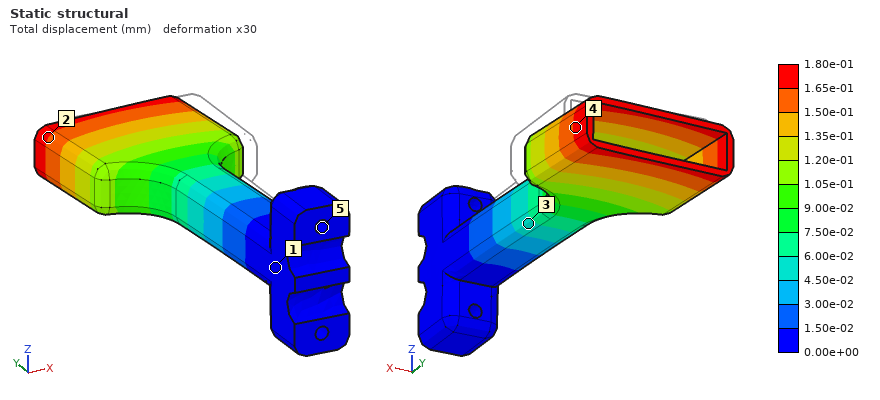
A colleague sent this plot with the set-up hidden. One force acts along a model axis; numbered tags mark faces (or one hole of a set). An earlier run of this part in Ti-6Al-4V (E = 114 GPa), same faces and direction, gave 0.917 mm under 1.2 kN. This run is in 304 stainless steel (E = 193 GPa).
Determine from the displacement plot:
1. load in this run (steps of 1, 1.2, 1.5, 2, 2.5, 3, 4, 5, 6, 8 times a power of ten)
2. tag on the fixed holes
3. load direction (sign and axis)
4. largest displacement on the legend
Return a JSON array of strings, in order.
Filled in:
["400 N", "5", "-X", "1.80e-01 mm"]
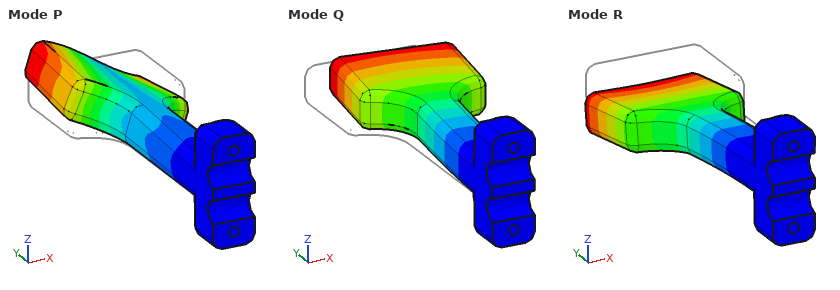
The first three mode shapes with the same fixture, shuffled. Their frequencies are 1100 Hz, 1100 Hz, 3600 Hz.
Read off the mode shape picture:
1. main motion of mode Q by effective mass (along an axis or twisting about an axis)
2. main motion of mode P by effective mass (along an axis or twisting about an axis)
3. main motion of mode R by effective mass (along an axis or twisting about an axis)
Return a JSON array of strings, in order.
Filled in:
["along X", "twisting about Y", "along Z"]
